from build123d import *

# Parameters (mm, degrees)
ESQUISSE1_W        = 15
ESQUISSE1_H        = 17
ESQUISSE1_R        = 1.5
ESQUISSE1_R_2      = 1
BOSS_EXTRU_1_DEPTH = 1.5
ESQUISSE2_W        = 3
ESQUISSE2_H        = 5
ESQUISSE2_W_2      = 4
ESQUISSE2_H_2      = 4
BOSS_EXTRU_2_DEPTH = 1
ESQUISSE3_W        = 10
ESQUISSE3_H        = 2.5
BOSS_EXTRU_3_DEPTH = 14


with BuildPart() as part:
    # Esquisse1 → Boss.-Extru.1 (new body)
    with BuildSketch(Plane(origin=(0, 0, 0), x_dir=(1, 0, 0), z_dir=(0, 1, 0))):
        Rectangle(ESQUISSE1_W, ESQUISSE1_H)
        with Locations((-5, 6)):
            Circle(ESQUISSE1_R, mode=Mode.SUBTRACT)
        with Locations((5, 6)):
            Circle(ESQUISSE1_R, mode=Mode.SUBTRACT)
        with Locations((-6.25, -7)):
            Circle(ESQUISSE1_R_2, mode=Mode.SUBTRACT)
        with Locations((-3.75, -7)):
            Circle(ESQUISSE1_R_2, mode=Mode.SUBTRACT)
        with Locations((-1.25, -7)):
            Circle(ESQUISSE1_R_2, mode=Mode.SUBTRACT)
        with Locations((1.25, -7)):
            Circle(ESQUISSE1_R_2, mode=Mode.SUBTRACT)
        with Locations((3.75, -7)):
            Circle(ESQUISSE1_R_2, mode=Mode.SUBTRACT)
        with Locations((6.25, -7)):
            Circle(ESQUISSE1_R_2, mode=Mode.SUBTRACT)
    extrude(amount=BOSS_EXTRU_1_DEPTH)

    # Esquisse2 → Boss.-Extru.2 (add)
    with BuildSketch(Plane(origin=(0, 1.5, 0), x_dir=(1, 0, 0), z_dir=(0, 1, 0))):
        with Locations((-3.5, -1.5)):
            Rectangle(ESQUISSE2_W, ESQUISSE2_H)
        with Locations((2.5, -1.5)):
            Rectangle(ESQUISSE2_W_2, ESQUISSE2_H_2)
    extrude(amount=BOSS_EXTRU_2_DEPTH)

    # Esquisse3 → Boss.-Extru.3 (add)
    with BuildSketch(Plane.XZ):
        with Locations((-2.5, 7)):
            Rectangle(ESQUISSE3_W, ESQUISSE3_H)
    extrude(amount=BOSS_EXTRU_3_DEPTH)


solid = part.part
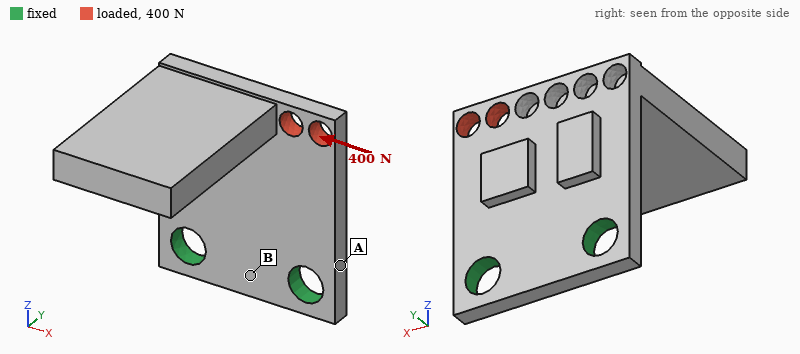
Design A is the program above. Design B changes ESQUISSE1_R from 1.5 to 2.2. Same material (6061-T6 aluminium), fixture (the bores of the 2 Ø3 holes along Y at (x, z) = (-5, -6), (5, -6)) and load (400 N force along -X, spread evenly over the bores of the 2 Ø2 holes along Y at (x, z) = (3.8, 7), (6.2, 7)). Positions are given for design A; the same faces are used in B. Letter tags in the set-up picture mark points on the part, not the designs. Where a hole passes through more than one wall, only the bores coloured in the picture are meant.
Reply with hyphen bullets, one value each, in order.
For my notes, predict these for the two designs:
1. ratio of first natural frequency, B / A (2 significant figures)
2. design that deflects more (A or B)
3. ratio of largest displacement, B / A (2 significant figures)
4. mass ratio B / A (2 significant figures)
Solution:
- 1.1
- A
- 0.91
- 0.97
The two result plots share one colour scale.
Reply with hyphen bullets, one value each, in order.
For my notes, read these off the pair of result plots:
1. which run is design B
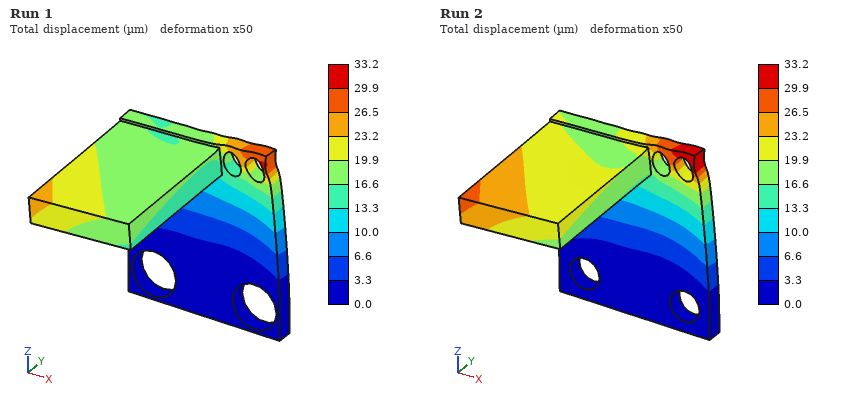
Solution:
- Run 1
